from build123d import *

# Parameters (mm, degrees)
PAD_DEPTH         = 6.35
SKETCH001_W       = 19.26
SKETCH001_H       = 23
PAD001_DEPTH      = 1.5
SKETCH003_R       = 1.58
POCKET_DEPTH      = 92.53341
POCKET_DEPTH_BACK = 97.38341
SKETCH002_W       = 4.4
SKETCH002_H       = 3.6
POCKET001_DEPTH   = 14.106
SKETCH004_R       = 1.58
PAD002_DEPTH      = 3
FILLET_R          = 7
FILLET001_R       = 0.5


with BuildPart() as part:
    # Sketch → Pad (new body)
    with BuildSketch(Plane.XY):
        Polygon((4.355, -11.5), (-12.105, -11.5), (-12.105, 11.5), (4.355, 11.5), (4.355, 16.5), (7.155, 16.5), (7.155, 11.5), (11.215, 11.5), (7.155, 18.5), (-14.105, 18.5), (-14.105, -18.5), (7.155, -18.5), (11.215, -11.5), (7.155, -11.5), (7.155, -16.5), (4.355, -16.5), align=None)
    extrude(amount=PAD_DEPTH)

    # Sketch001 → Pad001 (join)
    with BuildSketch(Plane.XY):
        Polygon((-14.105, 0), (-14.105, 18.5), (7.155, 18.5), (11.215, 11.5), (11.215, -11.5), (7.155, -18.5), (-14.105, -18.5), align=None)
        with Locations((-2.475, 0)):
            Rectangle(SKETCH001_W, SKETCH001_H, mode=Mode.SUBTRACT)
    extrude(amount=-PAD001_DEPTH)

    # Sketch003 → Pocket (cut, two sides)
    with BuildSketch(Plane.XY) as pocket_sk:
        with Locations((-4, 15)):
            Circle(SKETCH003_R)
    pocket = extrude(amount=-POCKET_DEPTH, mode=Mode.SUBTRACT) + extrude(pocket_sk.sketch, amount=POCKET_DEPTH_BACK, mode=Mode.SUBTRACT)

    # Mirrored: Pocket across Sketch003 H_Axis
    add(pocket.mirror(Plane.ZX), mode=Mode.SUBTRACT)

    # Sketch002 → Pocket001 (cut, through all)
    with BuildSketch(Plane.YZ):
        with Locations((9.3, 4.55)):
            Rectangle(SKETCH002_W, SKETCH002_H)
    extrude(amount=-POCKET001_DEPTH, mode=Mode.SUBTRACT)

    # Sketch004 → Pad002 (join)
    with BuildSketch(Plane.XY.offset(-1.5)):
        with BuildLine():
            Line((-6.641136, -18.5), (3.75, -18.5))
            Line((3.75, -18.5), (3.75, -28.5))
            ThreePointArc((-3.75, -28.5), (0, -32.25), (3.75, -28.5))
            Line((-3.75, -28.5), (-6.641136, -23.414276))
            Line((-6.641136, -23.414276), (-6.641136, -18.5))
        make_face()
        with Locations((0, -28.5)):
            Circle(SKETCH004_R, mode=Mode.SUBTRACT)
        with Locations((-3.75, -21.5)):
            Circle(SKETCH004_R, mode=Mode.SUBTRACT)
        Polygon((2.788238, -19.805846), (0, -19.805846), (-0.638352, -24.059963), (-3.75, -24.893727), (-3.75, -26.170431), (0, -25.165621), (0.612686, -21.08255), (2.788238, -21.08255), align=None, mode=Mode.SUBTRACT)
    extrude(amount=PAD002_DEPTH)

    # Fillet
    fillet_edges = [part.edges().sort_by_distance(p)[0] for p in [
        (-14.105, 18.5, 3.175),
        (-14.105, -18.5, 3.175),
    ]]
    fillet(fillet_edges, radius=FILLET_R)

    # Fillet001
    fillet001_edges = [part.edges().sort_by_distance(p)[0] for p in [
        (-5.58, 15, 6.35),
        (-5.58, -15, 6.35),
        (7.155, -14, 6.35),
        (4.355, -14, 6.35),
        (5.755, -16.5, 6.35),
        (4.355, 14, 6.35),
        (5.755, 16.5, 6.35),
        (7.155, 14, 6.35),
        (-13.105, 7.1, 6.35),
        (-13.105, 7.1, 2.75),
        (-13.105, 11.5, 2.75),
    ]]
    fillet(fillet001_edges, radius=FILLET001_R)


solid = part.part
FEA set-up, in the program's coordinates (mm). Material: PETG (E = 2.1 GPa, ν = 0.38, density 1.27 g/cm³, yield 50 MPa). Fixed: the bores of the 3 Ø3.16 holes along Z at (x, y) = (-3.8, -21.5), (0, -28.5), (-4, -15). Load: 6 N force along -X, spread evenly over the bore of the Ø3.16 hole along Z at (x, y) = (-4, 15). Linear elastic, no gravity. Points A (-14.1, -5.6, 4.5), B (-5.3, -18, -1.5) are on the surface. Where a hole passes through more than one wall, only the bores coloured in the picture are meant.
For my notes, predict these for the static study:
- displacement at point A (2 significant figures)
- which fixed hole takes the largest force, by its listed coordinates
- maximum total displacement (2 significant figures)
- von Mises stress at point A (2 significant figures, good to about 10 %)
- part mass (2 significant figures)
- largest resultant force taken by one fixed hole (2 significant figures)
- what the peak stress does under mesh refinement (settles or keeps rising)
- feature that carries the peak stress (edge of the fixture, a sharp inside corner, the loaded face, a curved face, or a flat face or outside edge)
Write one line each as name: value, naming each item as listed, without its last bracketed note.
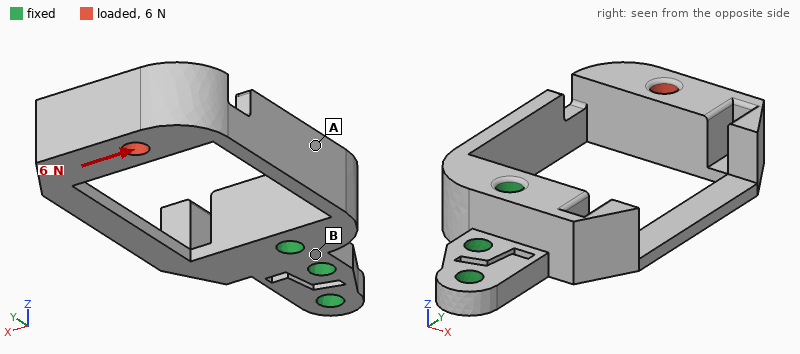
displacement at point A: 0.095 mm
which fixed hole takes the largest force, by its listed coordinates: (-4, -15)
maximum total displacement: 0.57 mm
von Mises stress at point A: 3.9 MPa
part mass: 3.6 g
largest resultant force taken by one fixed hole: 18 N
what the peak stress does under mesh refinement: keeps rising
feature that carries the peak stress: a sharp inside corner
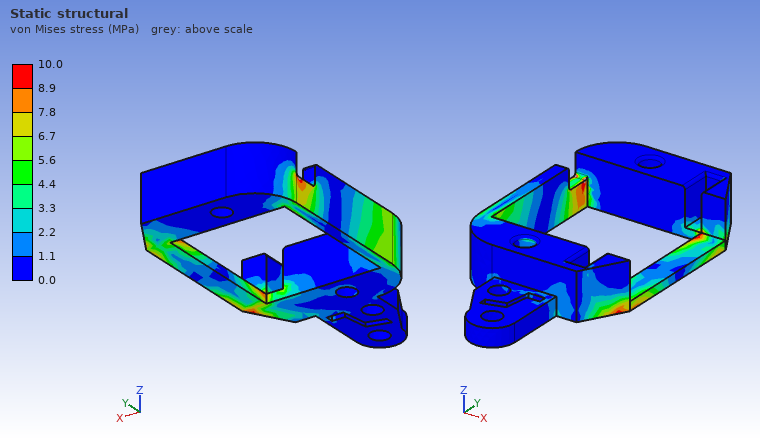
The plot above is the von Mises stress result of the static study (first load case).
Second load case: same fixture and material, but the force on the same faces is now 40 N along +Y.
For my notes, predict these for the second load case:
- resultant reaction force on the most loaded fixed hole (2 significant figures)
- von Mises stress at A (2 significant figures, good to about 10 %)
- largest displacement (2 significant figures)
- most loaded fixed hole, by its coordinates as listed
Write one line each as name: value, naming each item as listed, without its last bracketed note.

resultant reaction force on the most loaded fixed hole: 20 N
von Mises stress at A: 1.8 MPa
largest displacement: 0.55 mm
most loaded fixed hole, by its coordinates as listed: (-4, -15)
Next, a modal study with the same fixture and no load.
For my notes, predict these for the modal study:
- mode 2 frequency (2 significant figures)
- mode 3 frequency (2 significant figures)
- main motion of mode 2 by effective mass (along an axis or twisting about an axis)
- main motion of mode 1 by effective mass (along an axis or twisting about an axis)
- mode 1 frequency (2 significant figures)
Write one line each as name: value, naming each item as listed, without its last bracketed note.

mode 2 frequency: 450 Hz
mode 3 frequency: 950 Hz
main motion of mode 2 by effective mass: along X
main motion of mode 1 by effective mass: along Z
mode 1 frequency: 310 Hz
